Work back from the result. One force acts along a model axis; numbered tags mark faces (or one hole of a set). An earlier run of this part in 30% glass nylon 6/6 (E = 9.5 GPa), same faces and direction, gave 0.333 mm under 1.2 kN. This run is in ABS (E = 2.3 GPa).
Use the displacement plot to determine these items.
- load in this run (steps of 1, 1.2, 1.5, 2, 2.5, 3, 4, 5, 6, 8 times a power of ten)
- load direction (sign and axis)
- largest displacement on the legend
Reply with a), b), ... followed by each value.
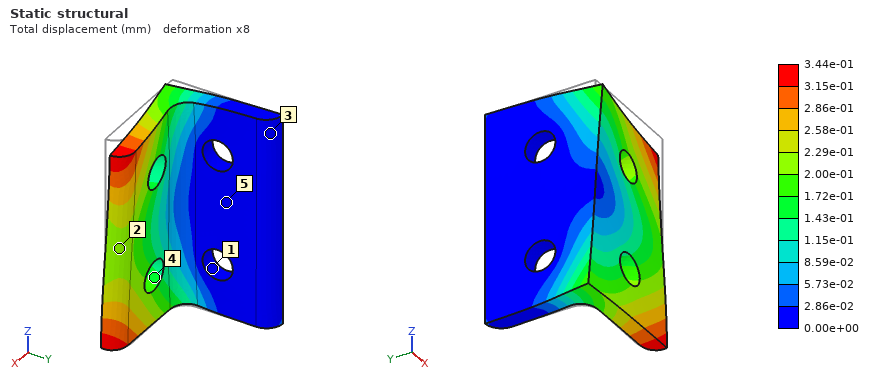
a) 300 N
b) -Z
c) 3.44e-01 mm
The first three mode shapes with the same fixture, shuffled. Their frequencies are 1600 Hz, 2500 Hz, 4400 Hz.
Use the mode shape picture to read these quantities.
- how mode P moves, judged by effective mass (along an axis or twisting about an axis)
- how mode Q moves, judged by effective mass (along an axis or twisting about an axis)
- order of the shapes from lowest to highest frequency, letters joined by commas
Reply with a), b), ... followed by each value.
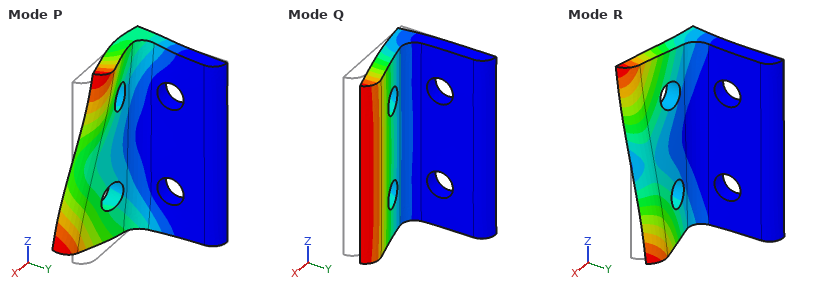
a) along Z
b) along Y
c) Q, R, P
